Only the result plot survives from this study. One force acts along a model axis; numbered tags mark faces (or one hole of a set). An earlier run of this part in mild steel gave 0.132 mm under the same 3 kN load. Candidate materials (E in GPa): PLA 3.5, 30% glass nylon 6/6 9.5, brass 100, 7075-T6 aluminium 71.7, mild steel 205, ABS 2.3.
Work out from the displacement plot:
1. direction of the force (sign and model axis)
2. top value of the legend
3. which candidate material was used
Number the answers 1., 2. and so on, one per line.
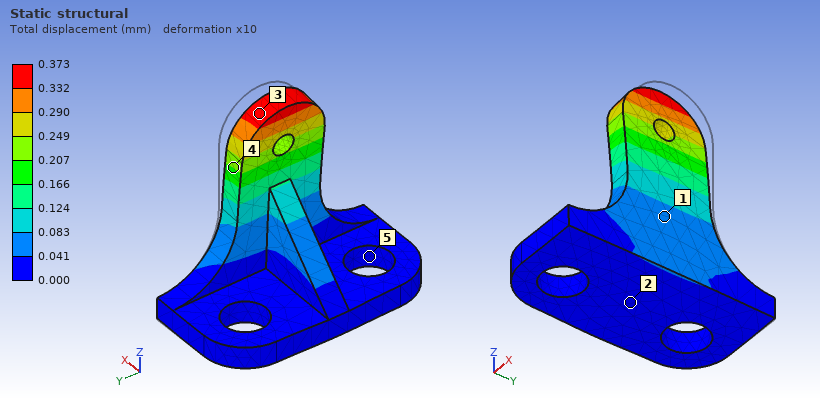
1. -X
2. 0.373 mm
3. 7075-T6 aluminium
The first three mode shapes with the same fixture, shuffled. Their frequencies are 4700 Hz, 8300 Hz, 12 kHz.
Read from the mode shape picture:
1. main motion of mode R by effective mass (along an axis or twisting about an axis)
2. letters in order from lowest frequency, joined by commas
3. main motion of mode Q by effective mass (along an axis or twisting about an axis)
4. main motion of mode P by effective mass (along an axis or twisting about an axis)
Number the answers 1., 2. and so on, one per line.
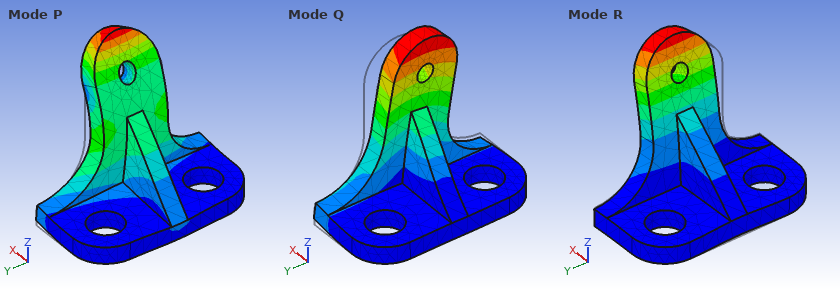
1. along X
2. R, Q, P
3. along Y
4. along Z
